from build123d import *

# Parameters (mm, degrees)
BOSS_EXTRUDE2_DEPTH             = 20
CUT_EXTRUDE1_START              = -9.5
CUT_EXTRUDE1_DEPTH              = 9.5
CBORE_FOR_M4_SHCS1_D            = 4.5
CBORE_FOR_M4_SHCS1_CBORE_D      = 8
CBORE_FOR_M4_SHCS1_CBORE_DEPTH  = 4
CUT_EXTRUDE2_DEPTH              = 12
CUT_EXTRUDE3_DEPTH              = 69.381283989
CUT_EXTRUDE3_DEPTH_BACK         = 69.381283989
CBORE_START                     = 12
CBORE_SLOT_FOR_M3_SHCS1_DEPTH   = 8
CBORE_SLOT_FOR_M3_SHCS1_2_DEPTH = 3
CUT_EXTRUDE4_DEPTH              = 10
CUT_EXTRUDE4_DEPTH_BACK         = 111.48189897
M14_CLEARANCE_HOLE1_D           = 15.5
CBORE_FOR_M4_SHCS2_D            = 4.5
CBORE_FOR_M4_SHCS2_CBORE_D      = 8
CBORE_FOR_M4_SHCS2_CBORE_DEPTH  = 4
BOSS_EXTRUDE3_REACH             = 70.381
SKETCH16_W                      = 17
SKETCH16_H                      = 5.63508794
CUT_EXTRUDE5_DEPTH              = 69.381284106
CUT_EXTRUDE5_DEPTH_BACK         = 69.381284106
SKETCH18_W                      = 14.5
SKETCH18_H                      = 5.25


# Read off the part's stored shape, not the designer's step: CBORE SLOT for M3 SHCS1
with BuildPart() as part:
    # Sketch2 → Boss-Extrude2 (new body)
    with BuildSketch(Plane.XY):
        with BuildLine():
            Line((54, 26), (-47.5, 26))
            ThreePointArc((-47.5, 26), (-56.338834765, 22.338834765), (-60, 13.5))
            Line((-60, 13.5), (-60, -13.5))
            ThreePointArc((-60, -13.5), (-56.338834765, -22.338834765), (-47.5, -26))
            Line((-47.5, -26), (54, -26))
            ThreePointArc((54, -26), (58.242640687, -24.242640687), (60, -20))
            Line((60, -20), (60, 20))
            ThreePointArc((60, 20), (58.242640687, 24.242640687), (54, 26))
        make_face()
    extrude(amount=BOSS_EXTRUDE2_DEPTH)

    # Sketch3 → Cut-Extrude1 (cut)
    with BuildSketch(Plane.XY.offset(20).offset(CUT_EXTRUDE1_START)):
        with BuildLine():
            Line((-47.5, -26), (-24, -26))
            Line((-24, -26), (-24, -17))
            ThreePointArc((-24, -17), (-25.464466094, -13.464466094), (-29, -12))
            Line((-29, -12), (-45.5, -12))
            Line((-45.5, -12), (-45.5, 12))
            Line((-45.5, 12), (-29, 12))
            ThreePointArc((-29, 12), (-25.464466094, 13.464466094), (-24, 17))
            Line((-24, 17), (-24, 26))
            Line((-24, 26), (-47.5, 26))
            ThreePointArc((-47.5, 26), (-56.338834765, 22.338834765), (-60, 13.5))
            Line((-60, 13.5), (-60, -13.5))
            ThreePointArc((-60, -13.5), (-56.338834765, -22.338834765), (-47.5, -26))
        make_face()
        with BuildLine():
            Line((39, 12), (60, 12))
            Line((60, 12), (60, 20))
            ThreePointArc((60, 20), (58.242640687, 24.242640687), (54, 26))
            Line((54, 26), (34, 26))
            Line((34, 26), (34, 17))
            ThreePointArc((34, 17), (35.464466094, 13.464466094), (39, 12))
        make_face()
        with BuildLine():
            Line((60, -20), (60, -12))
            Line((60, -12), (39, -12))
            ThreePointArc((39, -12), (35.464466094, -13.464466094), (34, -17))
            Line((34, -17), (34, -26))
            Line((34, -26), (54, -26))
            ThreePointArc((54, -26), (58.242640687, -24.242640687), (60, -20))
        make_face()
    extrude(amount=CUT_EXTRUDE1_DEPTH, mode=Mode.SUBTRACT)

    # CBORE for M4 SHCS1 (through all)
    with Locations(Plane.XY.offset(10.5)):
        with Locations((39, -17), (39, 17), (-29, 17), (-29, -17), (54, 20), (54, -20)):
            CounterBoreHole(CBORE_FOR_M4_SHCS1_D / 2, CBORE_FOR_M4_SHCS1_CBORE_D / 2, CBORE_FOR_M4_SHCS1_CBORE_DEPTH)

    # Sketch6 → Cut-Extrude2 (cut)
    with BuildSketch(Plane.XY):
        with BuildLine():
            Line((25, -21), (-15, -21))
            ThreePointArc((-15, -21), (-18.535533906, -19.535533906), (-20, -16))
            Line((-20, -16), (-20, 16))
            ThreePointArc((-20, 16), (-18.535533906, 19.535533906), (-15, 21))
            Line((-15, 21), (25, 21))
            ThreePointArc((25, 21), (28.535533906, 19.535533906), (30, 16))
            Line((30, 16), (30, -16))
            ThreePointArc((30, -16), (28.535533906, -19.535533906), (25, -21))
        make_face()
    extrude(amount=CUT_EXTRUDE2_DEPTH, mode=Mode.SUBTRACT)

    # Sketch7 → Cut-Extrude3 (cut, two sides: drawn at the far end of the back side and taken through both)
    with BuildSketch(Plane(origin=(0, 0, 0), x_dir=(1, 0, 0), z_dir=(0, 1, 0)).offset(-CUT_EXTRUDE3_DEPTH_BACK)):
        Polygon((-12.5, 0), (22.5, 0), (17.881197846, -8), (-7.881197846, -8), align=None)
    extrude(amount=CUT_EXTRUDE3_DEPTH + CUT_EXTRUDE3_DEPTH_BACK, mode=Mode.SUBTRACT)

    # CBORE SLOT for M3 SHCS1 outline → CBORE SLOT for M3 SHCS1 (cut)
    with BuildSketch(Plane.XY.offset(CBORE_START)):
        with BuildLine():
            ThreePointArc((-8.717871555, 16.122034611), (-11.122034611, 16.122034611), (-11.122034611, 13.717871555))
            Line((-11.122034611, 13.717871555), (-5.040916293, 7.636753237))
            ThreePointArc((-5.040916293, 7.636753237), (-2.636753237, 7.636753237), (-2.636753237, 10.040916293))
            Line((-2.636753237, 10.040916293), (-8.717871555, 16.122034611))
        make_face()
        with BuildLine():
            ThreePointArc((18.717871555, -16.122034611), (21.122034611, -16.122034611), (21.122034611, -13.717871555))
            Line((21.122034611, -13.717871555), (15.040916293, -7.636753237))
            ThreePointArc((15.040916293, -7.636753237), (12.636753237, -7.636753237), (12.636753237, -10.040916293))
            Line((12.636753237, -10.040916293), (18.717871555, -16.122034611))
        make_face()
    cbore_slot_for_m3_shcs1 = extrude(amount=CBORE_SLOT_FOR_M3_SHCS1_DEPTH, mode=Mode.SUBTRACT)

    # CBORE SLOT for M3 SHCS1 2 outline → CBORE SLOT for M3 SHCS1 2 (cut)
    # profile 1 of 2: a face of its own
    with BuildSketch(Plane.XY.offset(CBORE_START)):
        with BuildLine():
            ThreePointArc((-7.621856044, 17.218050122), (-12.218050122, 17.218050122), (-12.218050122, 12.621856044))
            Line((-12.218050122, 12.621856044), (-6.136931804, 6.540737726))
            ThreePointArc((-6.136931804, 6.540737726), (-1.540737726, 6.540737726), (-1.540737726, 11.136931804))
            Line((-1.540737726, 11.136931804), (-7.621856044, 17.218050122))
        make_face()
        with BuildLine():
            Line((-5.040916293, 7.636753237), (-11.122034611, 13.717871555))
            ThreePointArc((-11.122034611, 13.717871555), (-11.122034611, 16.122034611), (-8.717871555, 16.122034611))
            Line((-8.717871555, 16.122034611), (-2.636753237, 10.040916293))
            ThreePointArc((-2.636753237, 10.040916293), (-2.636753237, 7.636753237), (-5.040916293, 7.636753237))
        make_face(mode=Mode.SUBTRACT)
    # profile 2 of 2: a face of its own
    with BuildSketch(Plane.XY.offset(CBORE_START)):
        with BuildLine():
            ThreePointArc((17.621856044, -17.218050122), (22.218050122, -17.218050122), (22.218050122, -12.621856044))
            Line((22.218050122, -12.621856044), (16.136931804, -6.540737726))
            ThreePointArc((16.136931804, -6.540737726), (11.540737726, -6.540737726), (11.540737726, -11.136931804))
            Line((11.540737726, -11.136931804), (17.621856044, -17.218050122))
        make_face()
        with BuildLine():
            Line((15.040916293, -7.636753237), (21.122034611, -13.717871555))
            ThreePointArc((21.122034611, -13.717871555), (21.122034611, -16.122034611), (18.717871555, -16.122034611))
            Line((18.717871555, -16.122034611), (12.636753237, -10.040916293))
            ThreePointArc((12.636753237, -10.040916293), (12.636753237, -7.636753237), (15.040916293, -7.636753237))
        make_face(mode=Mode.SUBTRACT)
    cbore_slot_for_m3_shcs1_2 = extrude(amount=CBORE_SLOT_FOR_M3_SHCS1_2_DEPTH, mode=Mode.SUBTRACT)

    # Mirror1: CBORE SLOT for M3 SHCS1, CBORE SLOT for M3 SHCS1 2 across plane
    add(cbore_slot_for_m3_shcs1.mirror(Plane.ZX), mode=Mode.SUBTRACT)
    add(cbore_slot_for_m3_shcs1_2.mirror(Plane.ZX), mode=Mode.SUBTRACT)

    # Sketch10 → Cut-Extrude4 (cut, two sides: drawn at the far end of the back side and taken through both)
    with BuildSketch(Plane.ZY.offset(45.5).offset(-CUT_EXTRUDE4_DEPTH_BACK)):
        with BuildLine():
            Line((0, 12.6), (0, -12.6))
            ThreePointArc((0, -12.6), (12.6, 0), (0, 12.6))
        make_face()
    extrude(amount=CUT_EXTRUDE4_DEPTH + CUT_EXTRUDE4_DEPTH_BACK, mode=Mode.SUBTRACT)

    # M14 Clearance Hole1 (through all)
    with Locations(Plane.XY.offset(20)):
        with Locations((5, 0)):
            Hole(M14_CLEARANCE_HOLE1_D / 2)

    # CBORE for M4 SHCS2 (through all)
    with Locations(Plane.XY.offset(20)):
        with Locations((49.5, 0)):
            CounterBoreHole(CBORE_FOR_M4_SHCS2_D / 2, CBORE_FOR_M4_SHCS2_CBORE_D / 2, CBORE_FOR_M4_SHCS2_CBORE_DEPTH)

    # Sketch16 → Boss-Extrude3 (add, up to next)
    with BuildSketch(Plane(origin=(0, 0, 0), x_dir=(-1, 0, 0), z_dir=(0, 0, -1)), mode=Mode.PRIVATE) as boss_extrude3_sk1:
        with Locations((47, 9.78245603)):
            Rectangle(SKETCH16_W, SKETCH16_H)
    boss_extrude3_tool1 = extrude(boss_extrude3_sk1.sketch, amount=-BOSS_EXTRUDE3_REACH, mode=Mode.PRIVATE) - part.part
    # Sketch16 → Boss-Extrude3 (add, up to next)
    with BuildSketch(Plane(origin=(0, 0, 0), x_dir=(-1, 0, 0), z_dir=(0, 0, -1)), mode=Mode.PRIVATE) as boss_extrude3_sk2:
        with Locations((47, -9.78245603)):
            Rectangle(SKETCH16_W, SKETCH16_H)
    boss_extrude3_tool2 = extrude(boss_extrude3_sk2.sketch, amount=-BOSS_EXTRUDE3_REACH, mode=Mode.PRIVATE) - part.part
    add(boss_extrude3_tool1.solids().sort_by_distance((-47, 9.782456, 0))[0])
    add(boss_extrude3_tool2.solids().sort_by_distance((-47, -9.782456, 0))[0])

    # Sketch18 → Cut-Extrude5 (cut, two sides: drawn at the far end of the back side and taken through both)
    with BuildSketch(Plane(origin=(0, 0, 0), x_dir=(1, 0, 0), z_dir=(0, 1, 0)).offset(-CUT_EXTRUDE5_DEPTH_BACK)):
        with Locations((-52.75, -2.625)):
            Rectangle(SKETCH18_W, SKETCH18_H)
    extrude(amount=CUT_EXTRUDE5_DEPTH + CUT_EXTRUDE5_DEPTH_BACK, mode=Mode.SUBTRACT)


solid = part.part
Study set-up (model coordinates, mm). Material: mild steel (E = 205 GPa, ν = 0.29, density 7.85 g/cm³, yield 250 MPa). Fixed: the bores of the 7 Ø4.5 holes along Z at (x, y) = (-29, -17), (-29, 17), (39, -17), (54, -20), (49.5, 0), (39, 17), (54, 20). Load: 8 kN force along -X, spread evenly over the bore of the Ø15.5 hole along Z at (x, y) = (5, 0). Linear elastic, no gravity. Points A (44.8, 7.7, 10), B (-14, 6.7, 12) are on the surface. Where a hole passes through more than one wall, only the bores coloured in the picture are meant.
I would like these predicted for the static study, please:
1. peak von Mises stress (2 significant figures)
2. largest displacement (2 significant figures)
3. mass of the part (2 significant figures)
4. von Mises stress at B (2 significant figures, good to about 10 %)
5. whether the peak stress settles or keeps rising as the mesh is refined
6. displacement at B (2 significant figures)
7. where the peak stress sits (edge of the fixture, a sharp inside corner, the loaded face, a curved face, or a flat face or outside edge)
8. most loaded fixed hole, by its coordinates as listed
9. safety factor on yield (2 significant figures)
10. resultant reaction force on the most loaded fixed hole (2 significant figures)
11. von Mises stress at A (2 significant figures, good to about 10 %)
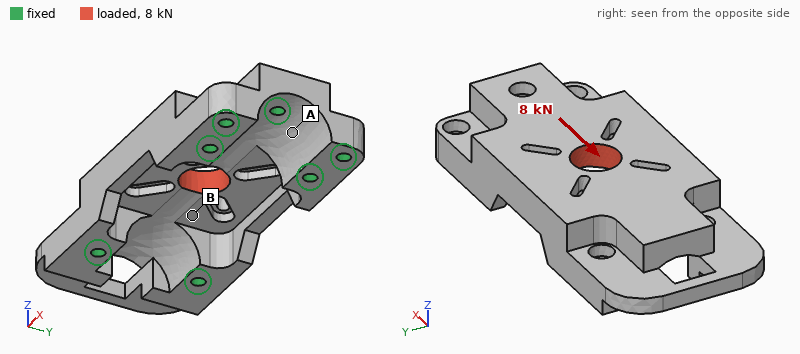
130 MPa
7.6 µm
420 g
22 MPa
settles
4.6 µm
a curved face
(49.5, 0)
2.0
2.0 kN
6.5 MPa
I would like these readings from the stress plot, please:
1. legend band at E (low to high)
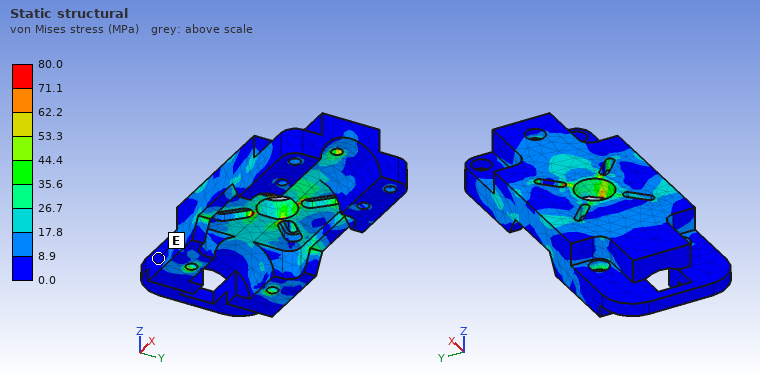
0.0 to 8.9 MPa
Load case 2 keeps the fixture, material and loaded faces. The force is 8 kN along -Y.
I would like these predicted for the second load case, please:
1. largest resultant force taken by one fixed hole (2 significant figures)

2.3 kN
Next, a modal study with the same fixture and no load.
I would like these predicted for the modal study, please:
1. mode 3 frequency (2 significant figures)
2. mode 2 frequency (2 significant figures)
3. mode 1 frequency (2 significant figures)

11 kHz
11 kHz
8700 Hz
